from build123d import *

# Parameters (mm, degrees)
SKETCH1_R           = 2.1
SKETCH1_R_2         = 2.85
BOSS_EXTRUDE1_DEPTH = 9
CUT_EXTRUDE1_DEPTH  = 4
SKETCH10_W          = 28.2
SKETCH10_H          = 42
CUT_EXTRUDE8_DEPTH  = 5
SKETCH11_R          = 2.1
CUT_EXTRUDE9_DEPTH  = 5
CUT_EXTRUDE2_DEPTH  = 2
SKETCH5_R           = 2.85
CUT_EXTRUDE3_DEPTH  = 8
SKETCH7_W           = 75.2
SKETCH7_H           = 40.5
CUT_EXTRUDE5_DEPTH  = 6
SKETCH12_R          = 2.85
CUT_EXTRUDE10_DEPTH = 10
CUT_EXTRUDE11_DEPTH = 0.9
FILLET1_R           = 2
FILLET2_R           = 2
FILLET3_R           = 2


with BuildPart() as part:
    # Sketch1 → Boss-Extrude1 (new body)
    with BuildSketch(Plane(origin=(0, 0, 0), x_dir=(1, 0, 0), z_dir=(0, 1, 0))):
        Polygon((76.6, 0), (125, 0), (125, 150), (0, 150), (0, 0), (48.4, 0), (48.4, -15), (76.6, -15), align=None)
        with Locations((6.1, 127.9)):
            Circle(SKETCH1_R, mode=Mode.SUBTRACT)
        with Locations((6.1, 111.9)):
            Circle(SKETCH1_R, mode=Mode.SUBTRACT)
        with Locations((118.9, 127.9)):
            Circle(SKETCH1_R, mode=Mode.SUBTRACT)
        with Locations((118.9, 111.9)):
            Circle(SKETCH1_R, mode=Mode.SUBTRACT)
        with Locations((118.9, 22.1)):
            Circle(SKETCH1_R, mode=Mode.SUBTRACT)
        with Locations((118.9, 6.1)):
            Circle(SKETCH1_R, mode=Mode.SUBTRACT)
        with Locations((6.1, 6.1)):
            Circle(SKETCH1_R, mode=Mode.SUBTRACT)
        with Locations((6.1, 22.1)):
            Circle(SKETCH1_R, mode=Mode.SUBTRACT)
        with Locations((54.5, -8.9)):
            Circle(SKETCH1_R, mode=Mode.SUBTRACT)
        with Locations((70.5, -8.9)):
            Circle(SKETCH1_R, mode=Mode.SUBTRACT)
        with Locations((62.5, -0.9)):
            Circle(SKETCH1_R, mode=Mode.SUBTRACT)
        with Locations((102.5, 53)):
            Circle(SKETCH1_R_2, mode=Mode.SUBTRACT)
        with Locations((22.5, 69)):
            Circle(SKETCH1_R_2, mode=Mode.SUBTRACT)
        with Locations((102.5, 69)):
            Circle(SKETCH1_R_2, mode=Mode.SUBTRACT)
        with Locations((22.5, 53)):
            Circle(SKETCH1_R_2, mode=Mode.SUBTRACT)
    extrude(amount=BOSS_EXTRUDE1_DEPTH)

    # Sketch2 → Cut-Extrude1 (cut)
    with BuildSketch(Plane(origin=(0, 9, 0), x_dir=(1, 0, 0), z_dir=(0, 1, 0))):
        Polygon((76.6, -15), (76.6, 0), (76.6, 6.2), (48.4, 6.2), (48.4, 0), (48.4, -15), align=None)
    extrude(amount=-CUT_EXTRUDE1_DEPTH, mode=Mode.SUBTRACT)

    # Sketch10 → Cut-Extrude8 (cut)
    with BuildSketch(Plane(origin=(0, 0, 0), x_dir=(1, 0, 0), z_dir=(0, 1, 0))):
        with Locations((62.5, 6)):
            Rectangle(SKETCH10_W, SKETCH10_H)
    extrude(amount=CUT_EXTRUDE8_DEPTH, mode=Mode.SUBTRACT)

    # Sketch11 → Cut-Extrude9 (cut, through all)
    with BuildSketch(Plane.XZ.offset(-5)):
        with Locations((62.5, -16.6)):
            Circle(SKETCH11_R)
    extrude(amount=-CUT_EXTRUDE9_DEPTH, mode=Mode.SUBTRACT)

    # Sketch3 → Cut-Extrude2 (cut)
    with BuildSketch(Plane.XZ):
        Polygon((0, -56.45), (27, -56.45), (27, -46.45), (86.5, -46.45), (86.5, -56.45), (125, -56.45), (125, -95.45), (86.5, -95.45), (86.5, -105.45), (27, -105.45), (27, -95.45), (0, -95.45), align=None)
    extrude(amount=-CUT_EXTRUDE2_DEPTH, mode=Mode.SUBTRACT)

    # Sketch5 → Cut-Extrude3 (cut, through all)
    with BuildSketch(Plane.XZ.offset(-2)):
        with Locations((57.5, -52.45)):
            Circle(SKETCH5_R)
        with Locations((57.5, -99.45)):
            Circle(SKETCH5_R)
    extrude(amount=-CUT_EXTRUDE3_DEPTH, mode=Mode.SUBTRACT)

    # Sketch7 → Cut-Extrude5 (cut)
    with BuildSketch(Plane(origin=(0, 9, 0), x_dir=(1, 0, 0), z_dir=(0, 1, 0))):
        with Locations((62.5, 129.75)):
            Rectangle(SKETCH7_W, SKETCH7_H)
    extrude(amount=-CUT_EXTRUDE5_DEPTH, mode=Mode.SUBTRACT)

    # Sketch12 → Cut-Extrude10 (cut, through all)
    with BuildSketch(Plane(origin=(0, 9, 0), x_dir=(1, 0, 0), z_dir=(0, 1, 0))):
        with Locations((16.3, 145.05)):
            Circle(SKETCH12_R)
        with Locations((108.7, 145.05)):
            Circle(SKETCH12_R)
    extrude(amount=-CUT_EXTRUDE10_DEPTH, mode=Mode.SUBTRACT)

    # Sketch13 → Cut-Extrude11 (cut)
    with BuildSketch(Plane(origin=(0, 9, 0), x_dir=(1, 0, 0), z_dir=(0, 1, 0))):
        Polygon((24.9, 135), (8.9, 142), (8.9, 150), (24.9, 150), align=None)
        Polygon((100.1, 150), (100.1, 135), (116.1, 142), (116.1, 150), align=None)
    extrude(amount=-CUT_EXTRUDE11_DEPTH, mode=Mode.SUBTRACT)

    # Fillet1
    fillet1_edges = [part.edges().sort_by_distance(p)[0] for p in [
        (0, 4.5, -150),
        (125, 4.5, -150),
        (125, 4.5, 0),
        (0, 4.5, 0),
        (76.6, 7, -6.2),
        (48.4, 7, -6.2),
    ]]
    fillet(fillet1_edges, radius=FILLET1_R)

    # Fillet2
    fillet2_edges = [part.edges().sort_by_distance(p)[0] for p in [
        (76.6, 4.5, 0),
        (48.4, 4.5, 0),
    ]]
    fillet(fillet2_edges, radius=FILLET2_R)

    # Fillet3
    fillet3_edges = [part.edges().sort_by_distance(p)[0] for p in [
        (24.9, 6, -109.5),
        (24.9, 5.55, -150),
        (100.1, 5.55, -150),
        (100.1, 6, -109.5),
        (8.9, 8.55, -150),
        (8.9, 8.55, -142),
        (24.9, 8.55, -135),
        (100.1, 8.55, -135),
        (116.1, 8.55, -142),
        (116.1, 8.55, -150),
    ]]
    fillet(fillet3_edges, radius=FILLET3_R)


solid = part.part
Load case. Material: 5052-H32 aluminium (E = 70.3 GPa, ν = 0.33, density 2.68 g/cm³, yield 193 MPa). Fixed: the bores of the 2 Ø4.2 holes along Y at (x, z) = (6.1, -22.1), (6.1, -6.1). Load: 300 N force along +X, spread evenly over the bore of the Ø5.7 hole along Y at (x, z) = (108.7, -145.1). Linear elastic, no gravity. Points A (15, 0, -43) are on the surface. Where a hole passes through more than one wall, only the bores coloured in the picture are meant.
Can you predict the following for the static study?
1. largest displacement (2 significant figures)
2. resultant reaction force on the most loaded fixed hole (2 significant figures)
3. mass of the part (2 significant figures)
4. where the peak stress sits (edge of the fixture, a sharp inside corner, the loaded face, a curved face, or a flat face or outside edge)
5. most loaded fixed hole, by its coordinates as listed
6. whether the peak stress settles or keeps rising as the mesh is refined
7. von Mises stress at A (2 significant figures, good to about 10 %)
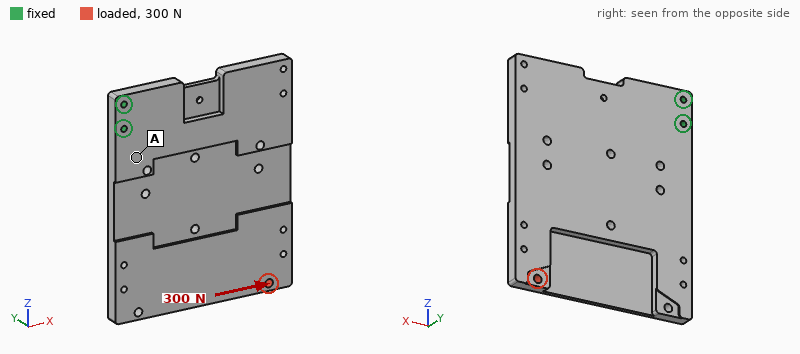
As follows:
0.11 mm
2.2 kN
350 g
edge of the fixture
(6.1, -22.1)
keeps rising
4.1 MPa
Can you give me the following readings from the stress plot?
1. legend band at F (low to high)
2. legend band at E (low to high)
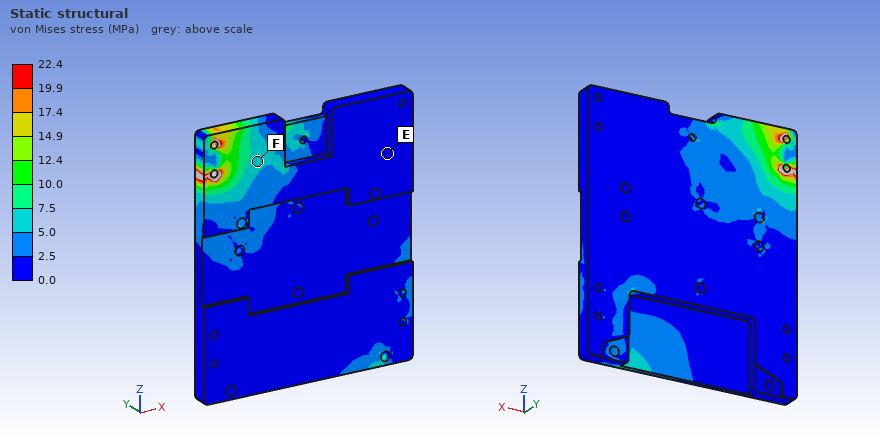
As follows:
5.0 to 7.5 MPa
0.0 to 2.5 MPa
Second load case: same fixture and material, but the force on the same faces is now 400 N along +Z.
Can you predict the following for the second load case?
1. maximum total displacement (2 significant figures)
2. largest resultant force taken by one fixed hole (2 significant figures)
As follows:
0.11 mm
2.2 kN
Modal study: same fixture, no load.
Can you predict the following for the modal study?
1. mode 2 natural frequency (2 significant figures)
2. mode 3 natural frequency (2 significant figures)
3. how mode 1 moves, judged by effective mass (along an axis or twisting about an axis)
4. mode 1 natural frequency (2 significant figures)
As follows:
450 Hz
740 Hz
along Y
240 Hz
